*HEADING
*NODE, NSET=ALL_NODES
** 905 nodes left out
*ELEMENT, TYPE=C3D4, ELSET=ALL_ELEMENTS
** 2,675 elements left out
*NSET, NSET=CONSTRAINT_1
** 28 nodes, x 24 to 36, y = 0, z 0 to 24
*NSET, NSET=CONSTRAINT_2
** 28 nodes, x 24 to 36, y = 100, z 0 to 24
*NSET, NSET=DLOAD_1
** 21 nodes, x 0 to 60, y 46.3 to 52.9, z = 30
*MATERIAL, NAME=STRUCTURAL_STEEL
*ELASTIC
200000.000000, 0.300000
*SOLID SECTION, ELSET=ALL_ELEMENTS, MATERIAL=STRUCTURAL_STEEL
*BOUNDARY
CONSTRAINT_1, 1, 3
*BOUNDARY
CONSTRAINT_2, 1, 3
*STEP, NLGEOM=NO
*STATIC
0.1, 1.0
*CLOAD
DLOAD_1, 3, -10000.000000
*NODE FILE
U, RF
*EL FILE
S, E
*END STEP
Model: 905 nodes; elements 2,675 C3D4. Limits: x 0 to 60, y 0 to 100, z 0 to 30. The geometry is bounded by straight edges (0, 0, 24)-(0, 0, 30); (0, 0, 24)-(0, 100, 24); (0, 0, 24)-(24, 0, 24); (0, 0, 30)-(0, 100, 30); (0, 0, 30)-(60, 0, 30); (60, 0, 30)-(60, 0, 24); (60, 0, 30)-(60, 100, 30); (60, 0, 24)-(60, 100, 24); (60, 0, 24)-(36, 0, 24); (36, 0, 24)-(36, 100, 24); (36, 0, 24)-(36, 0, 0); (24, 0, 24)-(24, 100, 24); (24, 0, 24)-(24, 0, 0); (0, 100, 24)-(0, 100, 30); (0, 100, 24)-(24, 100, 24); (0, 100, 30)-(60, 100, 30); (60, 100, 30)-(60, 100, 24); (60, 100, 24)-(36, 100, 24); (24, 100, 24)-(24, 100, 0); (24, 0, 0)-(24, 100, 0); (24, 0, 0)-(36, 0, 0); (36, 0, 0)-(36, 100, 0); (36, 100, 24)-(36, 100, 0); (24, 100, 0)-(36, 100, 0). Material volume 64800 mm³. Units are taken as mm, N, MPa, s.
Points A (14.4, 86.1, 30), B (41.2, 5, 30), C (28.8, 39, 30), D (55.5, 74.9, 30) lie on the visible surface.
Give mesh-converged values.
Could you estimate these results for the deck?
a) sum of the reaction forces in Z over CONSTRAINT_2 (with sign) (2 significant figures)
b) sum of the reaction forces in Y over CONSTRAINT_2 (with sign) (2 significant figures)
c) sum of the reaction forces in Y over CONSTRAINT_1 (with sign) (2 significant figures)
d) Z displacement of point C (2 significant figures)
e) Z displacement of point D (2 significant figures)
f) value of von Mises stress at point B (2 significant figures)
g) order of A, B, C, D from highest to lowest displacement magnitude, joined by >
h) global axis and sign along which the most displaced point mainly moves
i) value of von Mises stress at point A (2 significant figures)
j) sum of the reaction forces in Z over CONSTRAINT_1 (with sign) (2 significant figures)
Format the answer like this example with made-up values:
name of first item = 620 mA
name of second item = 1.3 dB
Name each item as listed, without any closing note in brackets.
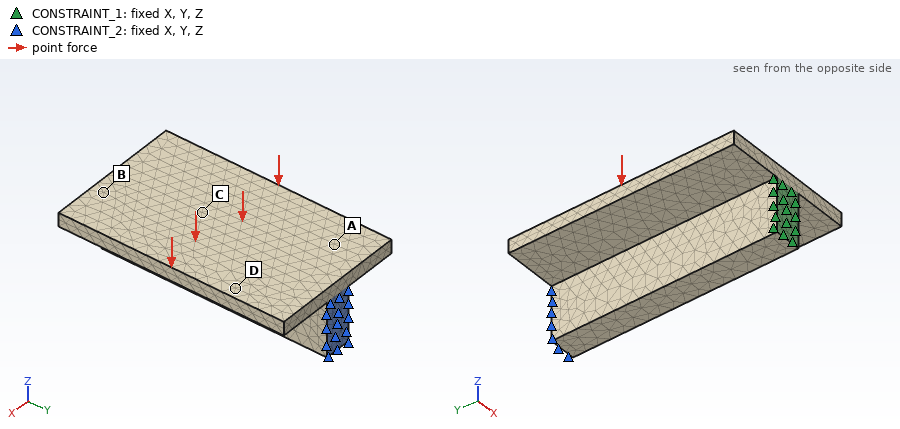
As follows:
sum of the reaction forces in Z over CONSTRAINT_2 (with sign) = 1.1e+05 N
sum of the reaction forces in Y over CONSTRAINT_2 (with sign) = -62000 N
sum of the reaction forces in Y over CONSTRAINT_1 (with sign) = 62000 N
Z displacement of point C = -0.33 mm
Z displacement of point D = -0.84 mm
value of von Mises stress at point B = 690 MPa
order of A, B, C, D from highest to lowest displacement magnitude, joined by > = D > C > A > B
global axis and sign along which the most displaced point mainly moves = -Z
value of von Mises stress at point A = 610 MPa
sum of the reaction forces in Z over CONSTRAINT_1 (with sign) = 1.0e+05 N
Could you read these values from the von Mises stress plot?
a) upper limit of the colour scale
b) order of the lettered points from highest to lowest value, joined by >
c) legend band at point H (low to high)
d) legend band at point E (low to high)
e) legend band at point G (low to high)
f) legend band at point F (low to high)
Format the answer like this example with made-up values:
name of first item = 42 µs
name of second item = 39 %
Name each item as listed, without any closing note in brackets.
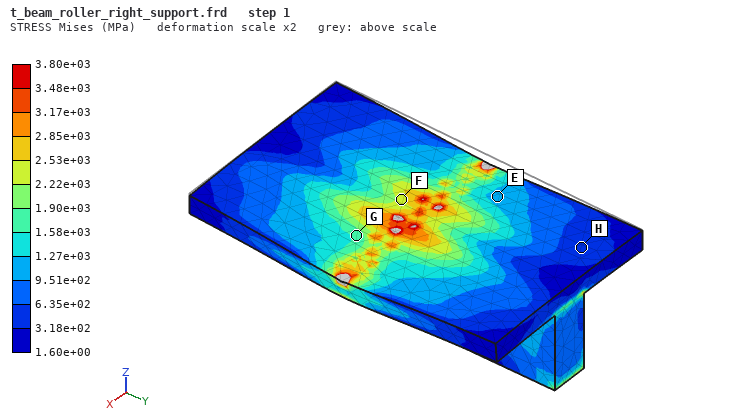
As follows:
upper limit of the colour scale = 3.80e+03 MPa
order of the lettered points from highest to lowest value, joined by > = F > G > E > H
legend band at point H = 3.18e+02 to 6.35e+02 MPa
legend band at point E = 9.51e+02 to 1.27e+03 MPa
legend band at point G = 1.58e+03 to 1.90e+03 MPa
legend band at point F = 2.22e+03 to 2.53e+03 MPa
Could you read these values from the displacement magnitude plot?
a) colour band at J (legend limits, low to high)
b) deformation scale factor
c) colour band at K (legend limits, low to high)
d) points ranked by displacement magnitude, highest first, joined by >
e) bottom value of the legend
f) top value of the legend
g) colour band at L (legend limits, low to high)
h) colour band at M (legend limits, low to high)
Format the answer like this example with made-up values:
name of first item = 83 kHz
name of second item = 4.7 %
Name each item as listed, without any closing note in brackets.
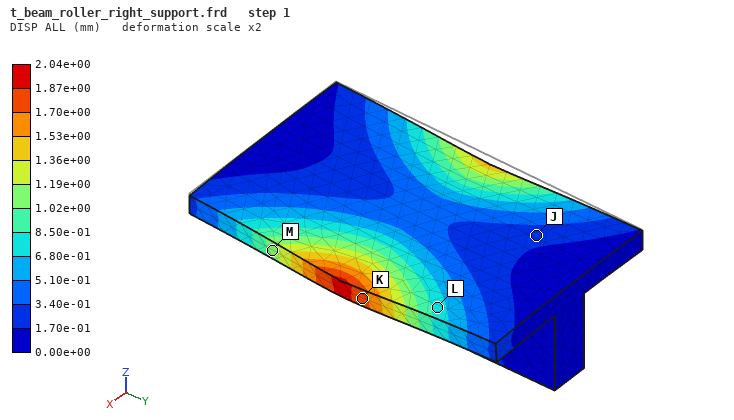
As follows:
colour band at J = 1.70e-01 to 3.40e-01 mm
deformation scale factor = 2
colour band at K = 1.70e+00 to 1.87e+00 mm
points ranked by displacement magnitude, highest first, joined by > = K > M > L > J
bottom value of the legend = 0.00e+00 mm
top value of the legend = 2.04e+00 mm
colour band at L = 6.80e-01 to 8.50e-01 mm
colour band at M = 1.02e+00 to 1.19e+00 mm
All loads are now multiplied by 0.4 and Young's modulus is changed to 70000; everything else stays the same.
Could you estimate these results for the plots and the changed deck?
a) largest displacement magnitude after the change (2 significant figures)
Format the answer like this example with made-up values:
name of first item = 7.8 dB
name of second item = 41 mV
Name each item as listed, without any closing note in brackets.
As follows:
largest displacement magnitude after the change = 2.3 mm
